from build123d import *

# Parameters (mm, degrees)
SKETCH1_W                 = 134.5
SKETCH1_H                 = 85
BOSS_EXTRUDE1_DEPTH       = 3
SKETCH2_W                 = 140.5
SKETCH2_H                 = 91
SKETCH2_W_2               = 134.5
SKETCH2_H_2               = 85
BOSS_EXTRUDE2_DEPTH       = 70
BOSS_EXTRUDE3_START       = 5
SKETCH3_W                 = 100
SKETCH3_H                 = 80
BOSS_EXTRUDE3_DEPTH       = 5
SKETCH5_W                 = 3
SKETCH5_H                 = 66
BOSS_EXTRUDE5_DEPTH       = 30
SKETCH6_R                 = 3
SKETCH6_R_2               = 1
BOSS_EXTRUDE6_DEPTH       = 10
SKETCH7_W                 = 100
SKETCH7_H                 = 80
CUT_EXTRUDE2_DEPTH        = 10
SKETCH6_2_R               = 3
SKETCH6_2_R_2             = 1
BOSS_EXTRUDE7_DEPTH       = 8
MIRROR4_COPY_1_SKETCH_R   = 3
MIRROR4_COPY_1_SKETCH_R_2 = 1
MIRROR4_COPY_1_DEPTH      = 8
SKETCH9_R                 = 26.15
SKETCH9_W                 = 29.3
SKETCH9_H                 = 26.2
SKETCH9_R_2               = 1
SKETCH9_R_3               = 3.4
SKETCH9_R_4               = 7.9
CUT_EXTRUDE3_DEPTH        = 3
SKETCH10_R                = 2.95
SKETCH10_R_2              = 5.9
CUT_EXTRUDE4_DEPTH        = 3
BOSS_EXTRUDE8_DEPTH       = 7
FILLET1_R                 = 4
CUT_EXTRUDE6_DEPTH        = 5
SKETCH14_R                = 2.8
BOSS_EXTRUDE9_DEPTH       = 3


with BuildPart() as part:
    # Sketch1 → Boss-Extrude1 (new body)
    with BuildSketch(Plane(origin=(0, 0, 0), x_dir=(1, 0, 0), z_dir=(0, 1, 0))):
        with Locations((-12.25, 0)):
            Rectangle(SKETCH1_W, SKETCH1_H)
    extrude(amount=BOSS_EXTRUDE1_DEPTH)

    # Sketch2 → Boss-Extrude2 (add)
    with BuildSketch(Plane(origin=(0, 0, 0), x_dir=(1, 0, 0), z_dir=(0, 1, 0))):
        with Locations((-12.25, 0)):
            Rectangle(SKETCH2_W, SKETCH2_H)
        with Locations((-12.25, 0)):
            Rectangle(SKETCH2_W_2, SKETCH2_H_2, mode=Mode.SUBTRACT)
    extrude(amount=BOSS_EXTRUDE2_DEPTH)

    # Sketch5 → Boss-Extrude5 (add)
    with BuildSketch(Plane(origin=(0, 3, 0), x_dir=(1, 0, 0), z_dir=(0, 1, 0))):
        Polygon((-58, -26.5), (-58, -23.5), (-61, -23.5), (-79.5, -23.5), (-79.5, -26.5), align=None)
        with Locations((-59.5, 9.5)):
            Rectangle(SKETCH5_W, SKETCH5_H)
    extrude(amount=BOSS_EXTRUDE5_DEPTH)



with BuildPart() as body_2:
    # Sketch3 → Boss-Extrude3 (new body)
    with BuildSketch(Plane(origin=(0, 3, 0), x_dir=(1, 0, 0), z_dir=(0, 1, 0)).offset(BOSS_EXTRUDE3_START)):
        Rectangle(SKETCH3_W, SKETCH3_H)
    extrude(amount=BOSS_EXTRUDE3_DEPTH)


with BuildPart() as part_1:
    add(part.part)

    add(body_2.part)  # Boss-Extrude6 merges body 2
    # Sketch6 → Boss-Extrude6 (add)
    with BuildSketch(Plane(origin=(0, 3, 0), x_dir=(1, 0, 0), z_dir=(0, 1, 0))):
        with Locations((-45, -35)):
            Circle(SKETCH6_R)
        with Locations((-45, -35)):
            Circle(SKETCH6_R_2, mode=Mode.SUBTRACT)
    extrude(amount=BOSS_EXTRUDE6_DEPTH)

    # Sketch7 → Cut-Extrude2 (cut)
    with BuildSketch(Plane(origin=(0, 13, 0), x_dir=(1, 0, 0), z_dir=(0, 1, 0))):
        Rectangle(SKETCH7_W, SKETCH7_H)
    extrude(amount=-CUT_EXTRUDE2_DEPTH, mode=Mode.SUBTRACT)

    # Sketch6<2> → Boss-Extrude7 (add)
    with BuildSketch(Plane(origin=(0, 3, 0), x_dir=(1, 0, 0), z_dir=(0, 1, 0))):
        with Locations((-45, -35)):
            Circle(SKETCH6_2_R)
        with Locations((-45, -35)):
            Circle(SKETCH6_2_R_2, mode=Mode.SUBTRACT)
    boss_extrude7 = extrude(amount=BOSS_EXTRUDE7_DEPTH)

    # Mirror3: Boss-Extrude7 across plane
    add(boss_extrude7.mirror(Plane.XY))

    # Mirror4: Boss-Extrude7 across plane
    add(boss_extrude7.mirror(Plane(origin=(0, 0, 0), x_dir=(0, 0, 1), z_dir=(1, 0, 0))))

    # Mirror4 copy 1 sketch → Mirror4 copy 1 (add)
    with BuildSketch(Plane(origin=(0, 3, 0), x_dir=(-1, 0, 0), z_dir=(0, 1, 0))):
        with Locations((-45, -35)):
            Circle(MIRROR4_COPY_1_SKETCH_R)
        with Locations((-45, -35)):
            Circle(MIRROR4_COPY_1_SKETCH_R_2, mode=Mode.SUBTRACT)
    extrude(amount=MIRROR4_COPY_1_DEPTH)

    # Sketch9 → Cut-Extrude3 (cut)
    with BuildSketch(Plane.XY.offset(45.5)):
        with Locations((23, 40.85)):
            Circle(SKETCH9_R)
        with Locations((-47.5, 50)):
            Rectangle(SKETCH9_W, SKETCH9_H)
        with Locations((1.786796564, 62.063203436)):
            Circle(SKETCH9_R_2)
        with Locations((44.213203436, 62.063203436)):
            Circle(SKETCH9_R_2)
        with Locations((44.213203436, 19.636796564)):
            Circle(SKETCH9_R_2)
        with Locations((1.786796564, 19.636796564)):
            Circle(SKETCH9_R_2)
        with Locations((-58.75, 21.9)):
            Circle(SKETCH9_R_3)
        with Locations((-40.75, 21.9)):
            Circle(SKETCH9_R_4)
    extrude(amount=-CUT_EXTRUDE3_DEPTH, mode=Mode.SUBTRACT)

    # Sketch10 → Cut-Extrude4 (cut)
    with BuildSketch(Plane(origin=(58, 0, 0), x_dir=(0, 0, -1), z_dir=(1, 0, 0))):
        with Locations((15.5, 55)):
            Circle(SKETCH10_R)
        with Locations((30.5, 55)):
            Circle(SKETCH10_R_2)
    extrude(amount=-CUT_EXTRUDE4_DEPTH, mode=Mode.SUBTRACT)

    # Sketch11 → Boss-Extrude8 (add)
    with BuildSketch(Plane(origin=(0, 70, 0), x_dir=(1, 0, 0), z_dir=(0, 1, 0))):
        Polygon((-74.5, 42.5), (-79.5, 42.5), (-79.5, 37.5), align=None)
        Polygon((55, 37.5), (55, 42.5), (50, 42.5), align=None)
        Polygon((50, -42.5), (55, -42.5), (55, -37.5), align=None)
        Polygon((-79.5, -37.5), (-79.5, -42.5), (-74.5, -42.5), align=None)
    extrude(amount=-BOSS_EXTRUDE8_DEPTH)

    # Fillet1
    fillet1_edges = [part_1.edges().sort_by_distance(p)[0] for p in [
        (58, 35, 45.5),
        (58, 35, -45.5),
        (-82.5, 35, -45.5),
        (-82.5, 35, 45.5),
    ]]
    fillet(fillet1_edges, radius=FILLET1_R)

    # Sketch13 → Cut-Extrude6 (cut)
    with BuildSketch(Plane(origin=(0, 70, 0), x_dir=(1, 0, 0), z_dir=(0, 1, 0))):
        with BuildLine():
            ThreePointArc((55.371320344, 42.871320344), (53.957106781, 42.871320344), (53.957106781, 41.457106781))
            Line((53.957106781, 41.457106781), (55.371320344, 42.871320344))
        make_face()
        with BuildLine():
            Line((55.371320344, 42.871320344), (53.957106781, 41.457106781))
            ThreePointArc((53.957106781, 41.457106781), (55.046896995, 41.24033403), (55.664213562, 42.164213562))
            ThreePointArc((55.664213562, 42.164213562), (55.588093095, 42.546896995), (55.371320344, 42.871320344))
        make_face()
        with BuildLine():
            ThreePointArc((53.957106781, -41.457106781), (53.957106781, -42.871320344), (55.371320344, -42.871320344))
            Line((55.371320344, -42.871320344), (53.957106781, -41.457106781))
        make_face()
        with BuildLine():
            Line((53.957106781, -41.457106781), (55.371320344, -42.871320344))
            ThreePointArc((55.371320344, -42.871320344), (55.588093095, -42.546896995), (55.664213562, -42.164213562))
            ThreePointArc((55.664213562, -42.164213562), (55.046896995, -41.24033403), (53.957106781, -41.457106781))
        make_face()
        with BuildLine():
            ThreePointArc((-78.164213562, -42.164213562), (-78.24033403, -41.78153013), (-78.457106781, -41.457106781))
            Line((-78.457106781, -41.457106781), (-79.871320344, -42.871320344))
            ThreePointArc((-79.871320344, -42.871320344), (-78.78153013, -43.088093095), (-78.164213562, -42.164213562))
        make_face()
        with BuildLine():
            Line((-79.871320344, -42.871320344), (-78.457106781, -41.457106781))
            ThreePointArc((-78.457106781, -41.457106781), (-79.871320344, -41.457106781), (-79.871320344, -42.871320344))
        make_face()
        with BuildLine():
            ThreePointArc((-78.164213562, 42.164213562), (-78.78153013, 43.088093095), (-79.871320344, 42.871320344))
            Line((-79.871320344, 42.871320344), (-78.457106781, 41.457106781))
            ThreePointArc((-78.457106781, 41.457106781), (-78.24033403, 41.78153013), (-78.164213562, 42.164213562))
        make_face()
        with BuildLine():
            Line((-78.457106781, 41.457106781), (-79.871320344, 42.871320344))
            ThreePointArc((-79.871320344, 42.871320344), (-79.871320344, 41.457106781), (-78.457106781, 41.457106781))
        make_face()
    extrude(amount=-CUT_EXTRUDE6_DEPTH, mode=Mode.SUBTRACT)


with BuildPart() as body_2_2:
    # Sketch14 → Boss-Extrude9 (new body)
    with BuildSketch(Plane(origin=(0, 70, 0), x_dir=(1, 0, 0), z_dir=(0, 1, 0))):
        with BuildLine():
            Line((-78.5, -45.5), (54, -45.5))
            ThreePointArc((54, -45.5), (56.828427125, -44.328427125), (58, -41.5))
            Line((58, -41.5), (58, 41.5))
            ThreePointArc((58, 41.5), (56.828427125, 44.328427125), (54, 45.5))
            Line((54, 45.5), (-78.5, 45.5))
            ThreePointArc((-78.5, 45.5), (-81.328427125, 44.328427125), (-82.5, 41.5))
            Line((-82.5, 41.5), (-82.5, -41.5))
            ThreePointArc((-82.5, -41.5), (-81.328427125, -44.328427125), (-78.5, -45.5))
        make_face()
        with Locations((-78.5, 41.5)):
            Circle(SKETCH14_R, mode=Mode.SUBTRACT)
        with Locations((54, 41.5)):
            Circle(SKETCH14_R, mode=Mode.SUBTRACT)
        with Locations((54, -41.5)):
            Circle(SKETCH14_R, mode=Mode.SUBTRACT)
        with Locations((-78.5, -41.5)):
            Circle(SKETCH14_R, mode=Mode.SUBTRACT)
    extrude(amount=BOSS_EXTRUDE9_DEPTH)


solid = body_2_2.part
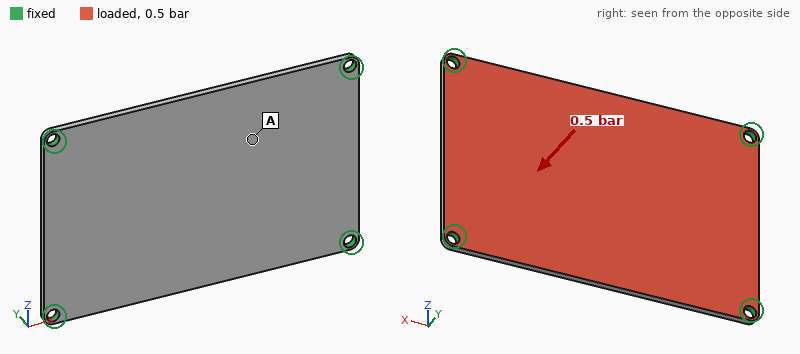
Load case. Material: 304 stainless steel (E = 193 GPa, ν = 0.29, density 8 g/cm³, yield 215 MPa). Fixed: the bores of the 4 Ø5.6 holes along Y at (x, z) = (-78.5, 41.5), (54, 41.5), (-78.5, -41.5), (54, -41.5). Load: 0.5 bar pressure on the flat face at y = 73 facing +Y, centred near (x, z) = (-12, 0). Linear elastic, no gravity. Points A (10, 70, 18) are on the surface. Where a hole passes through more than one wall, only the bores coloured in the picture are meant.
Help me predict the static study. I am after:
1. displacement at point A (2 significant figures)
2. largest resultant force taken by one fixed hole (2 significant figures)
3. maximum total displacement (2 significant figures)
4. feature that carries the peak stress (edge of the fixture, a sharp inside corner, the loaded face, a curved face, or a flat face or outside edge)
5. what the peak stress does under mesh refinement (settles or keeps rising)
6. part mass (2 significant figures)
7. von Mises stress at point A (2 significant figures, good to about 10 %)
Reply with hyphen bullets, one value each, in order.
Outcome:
- 0.12 mm
- 160 N
- 0.15 mm
- edge of the fixture
- keeps rising
- 300 g
- 21 MPa
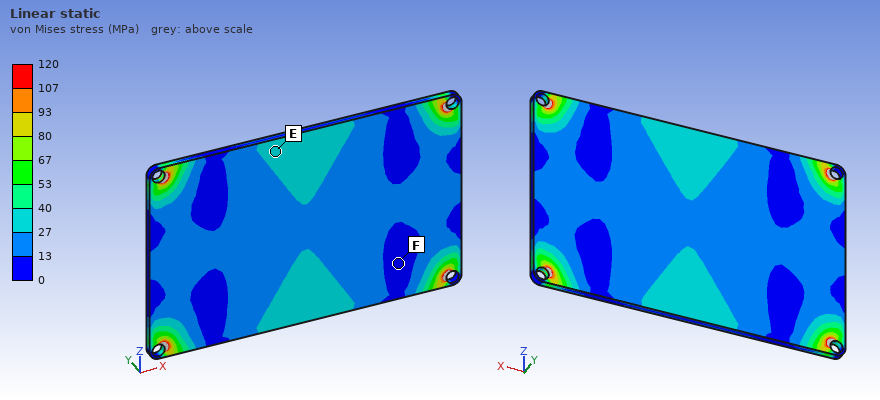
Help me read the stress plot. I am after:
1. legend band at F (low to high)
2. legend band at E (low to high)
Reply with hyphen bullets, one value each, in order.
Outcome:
- 0 to 13 MPa
- 27 to 40 MPa
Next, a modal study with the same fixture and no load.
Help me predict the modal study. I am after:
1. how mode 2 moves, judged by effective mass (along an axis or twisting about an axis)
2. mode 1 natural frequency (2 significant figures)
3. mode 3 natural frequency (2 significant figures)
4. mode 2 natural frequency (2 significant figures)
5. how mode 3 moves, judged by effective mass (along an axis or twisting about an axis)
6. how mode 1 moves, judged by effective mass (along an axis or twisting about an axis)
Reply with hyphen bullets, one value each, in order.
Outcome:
- twisting about X
- 690 Hz
- 1800 Hz
- 1200 Hz
- twisting about Z
- along Y
